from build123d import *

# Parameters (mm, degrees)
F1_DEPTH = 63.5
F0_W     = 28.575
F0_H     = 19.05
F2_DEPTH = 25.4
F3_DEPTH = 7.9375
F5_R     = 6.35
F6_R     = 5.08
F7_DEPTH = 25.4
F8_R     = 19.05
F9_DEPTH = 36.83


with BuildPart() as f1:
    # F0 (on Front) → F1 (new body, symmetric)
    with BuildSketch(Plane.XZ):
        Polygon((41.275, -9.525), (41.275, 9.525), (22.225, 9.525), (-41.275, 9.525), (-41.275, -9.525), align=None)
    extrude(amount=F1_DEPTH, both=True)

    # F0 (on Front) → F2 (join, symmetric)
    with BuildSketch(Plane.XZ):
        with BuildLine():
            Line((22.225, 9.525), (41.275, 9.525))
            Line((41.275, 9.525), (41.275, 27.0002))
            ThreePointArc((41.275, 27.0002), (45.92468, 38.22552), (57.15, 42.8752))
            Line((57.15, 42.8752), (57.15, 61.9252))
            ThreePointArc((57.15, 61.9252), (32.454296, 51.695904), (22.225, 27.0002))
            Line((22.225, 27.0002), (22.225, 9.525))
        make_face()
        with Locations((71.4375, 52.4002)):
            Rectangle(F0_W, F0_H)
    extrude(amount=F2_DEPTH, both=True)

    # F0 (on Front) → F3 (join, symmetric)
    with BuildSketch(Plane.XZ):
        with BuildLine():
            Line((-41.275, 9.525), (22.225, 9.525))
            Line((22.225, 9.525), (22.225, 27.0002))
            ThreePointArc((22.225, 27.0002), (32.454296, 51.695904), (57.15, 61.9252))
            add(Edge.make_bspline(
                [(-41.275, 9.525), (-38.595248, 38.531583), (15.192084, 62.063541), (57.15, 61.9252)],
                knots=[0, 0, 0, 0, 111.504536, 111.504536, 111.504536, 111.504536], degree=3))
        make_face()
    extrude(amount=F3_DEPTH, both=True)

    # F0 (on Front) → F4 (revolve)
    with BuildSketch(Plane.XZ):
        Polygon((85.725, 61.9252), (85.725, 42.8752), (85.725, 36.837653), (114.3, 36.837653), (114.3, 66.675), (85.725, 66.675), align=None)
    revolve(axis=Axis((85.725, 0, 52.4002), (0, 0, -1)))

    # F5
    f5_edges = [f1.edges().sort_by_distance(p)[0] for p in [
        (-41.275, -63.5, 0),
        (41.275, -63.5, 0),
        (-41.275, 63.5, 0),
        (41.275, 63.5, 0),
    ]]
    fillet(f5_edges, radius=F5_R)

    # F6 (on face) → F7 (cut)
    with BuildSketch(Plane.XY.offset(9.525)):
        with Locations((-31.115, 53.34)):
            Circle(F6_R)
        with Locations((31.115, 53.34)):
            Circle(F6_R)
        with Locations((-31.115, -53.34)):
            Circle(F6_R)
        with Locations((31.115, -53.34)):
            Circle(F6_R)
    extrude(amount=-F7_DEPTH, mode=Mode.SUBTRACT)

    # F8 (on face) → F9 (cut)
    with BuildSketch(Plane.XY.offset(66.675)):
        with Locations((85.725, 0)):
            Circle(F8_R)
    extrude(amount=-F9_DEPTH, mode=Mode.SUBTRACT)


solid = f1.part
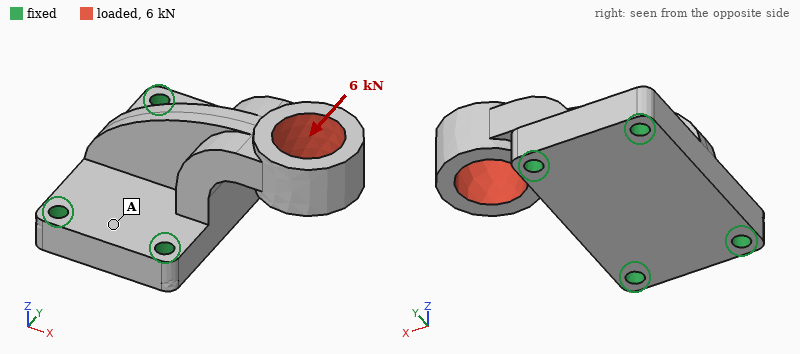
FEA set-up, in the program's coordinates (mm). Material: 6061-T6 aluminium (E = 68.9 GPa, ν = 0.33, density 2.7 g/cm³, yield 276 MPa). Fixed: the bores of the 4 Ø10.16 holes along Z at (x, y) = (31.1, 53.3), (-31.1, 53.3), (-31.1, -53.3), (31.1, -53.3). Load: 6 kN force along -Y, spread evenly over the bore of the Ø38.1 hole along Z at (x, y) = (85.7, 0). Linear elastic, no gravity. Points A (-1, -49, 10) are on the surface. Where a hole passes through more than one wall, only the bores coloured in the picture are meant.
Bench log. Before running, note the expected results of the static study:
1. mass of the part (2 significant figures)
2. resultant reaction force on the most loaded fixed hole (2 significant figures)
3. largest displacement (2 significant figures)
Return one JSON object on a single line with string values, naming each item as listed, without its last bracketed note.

{"mass of the part": "900 g", "resultant reaction force on the most loaded fixed hole": "4.9 kN", "largest displacement": "0.39 mm"}
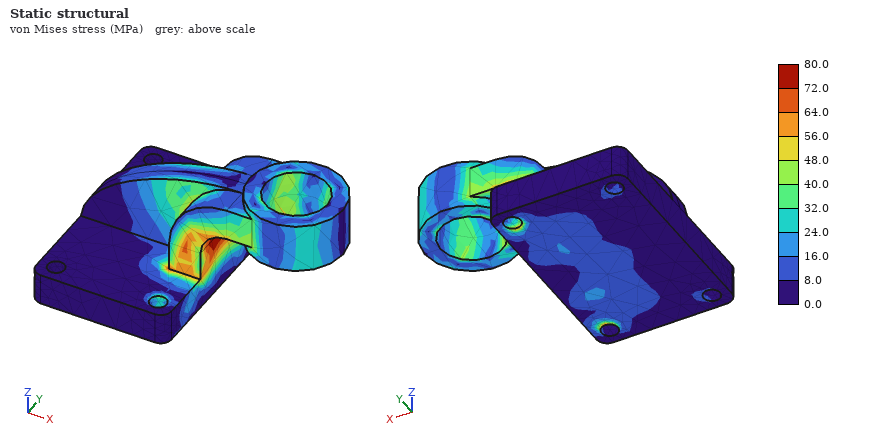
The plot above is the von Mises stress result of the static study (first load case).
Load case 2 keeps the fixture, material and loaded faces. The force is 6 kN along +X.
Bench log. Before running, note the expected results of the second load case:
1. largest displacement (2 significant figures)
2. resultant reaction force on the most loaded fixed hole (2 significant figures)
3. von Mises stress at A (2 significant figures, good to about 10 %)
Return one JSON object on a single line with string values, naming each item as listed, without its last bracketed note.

{"largest displacement": "0.14 mm", "resultant reaction force on the most loaded fixed hole": "3.3 kN", "von Mises stress at A": "9.0 MPa"}
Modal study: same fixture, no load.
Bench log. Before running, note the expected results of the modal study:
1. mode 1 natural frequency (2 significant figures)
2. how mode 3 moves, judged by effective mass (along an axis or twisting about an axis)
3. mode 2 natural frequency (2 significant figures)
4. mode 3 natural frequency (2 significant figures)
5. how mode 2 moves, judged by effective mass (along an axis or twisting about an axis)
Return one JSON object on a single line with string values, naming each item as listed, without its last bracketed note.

{"mode 1 natural frequency": "1800 Hz", "how mode 3 moves, judged by effective mass": "along X", "mode 2 natural frequency": "2000 Hz", "mode 3 natural frequency": "3900 Hz", "how mode 2 moves, judged by effective mass": "along Y"}
